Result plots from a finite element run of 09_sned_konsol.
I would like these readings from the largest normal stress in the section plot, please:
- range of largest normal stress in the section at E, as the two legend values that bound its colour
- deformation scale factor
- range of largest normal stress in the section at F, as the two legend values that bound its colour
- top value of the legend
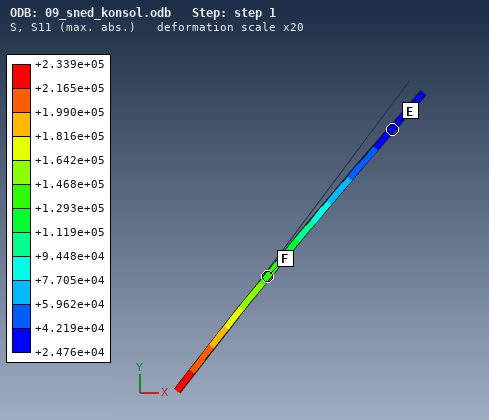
+2.476e+04 to +4.219e+04
20
+1.293e+05 to +1.468e+05
+2.339e+05
